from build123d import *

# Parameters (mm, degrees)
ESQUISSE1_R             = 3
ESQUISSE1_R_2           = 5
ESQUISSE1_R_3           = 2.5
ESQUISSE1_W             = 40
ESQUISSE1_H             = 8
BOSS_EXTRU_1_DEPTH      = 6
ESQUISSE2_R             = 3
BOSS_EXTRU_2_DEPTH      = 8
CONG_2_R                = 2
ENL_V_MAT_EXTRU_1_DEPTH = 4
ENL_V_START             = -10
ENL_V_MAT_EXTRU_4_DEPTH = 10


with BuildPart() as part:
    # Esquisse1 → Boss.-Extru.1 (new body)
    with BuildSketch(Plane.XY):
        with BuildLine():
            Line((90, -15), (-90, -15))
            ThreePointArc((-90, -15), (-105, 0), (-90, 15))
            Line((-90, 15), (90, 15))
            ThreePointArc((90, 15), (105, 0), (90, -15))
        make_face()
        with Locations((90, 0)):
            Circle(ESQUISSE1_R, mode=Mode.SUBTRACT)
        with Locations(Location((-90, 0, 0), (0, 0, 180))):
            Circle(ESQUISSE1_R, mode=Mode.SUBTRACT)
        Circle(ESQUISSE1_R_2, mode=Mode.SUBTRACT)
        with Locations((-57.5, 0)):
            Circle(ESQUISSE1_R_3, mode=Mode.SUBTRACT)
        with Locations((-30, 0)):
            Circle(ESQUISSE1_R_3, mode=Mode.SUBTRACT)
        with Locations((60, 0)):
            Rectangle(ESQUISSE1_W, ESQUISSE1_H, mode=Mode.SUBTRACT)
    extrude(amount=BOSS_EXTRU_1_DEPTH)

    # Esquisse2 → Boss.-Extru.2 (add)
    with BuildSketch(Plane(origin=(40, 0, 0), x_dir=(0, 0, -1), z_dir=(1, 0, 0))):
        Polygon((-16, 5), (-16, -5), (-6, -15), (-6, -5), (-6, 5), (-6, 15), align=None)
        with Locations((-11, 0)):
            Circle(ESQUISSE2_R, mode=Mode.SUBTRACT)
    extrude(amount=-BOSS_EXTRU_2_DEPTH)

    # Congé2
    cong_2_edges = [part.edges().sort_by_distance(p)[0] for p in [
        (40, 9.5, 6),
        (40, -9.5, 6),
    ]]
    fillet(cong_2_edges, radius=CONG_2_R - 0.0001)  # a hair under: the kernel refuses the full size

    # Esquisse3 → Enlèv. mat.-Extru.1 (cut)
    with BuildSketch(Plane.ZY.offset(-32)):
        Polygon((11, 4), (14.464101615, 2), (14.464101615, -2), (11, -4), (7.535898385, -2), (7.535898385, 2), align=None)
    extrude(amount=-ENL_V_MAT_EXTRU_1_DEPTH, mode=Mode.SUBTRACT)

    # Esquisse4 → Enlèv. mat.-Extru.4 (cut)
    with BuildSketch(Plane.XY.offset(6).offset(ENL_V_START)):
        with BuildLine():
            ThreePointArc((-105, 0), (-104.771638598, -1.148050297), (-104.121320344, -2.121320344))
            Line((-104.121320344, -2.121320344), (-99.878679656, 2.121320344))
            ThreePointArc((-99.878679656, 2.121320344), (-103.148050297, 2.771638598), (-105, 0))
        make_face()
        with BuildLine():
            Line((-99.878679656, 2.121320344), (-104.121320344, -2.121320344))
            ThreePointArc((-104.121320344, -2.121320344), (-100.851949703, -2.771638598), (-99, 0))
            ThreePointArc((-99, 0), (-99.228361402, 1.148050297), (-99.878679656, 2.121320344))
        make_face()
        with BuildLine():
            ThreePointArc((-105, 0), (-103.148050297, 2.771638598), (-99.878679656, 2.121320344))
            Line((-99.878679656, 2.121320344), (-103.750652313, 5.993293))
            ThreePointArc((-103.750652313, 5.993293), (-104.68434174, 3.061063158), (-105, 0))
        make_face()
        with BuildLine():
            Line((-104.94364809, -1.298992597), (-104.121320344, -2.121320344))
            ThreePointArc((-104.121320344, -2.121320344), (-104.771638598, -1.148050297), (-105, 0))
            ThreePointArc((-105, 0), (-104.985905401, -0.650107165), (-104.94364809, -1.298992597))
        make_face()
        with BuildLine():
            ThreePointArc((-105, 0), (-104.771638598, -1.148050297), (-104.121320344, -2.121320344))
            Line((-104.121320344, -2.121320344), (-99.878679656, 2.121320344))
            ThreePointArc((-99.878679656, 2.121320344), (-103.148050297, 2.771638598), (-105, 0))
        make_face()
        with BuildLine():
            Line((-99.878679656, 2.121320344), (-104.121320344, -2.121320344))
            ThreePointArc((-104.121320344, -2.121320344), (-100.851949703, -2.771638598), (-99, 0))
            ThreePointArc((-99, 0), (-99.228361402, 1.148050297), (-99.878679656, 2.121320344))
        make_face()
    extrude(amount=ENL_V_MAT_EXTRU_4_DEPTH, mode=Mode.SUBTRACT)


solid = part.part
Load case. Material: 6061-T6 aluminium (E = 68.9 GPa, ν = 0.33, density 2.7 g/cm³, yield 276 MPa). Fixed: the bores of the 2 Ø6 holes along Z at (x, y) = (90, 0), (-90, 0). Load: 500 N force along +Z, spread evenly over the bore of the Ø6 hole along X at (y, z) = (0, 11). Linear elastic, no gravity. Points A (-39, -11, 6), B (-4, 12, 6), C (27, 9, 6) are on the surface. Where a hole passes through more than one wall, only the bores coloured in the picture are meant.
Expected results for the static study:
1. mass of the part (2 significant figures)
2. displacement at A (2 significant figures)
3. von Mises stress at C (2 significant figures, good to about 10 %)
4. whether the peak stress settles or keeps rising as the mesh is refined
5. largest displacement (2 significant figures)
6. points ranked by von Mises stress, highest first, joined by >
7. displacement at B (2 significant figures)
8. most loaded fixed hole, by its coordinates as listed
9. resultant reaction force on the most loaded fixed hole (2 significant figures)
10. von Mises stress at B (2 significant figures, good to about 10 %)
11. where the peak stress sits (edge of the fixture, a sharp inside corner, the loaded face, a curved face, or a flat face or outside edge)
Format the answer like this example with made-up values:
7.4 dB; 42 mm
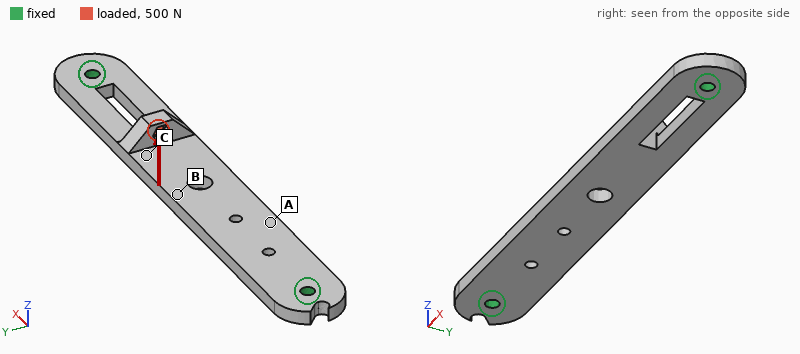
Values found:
94 g; 0.14 mm; 38 MPa; keeps rising; 0.30 mm; C > B > A; 0.28 mm; (90, 0); 390 N; 26 MPa; edge of the fixture
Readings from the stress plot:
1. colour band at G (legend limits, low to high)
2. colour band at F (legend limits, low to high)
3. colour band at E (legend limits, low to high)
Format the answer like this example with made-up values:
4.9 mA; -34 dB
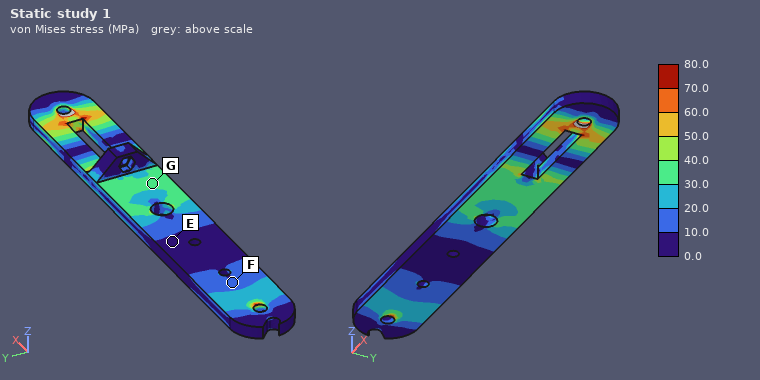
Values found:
30.0 to 40.0 MPa; 10.0 to 20.0 MPa; 0.0 to 10.0 MPa
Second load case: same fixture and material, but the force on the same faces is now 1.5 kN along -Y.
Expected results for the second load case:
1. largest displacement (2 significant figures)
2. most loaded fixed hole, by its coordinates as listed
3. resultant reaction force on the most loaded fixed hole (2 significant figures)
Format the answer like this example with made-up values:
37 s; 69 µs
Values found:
0.30 mm; (90, 0); 1.0 kN
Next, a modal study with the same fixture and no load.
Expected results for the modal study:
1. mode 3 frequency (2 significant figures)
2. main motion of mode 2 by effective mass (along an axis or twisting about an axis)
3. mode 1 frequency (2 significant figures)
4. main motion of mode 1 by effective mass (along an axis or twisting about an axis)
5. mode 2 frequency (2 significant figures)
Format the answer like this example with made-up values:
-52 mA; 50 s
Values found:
2500 Hz; along Y; 910 Hz; along Z; 2400 Hz
